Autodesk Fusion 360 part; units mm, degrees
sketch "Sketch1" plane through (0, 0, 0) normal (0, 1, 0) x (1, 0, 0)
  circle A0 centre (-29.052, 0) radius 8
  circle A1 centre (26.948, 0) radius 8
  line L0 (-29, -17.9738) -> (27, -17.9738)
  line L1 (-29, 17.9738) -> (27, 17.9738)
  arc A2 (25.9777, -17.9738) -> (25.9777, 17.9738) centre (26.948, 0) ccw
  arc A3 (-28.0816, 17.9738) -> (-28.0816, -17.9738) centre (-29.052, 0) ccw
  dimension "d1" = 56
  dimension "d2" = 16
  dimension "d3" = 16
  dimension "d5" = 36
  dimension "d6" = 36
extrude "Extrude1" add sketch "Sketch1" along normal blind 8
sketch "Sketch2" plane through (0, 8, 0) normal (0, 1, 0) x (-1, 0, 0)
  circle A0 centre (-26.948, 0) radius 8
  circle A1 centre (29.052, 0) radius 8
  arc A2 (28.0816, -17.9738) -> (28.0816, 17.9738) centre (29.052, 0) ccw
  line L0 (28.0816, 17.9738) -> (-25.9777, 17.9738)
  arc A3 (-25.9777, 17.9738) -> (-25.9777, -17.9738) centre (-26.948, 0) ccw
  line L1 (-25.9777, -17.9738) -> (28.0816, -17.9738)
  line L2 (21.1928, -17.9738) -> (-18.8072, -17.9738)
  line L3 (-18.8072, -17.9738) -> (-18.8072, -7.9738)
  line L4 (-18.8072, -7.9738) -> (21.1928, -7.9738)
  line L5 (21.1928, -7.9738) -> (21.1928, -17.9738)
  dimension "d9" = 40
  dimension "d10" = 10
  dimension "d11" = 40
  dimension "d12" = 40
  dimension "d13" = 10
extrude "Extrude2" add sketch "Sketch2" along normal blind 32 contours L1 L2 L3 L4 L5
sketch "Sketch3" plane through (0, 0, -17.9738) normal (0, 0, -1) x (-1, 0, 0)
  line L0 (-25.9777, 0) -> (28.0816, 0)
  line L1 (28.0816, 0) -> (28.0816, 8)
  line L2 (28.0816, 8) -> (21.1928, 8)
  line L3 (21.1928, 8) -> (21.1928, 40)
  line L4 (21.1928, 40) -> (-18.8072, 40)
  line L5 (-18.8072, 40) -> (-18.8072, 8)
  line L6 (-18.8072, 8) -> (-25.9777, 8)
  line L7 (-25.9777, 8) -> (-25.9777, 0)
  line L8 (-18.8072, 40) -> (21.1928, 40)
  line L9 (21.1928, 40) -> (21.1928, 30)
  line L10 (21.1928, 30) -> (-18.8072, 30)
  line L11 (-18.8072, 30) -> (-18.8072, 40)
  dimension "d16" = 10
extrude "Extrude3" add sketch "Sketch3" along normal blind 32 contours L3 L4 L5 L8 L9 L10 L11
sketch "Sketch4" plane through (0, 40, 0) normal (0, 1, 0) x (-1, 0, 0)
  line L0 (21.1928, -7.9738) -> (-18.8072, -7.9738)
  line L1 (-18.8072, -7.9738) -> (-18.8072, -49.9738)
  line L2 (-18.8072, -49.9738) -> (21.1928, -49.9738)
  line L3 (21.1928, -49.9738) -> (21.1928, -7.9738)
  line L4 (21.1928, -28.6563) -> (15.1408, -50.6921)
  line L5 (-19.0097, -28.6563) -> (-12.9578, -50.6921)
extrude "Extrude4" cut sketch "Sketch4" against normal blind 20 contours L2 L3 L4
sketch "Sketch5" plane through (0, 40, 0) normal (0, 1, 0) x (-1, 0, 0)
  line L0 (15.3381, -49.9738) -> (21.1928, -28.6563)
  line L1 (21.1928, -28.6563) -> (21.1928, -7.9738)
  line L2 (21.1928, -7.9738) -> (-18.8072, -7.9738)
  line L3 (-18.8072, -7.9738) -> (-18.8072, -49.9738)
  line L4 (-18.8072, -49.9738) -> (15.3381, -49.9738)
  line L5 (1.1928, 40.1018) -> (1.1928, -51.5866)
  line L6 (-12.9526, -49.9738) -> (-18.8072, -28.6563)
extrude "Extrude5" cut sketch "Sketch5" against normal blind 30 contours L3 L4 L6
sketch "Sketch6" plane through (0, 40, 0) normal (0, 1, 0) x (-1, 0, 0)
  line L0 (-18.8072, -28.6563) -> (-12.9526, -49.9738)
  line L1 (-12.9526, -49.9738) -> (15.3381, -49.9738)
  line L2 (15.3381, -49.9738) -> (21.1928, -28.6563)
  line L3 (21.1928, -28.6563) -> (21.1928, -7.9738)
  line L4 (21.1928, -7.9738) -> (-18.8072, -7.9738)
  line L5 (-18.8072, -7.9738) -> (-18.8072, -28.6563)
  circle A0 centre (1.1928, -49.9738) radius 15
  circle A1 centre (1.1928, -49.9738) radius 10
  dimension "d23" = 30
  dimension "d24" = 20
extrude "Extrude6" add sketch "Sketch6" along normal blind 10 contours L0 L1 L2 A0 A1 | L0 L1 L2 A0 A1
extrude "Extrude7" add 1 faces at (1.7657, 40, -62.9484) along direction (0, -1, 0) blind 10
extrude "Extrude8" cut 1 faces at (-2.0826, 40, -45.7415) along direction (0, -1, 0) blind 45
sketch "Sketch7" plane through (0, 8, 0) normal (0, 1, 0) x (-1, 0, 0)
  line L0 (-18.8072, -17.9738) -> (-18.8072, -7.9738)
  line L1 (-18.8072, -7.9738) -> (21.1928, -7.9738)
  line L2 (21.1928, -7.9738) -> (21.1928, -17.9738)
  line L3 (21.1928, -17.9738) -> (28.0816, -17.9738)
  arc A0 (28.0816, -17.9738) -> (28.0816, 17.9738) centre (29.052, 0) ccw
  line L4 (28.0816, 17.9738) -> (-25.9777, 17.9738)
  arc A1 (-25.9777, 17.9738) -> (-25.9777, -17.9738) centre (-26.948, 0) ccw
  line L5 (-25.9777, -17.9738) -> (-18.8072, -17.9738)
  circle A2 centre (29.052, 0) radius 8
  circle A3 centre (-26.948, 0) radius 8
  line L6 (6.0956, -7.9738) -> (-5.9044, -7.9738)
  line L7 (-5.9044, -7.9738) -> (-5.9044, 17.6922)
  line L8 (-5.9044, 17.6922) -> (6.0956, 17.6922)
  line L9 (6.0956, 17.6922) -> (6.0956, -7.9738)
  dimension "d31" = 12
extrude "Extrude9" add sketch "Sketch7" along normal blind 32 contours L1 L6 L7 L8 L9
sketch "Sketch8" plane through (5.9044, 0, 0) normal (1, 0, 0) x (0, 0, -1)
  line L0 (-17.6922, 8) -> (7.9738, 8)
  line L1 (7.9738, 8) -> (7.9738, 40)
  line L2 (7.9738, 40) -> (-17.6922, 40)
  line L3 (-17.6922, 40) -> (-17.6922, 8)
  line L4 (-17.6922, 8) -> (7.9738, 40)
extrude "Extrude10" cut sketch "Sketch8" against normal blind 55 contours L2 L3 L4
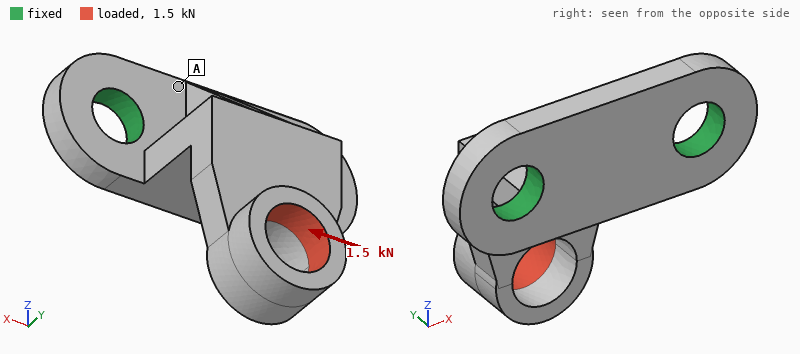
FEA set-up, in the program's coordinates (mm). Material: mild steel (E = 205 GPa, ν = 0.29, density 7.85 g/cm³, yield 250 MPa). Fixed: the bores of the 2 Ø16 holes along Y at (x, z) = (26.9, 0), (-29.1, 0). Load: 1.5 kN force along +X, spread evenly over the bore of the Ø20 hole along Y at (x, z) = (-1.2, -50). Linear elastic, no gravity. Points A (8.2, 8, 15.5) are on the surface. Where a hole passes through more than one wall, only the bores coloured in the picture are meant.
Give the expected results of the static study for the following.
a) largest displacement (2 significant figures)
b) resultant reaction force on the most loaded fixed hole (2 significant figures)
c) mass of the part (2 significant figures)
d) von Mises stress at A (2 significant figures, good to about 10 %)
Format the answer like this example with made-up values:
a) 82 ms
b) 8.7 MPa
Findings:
a) 55 µm
b) 2.1 kN
c) 430 g
d) 5.4 MPa
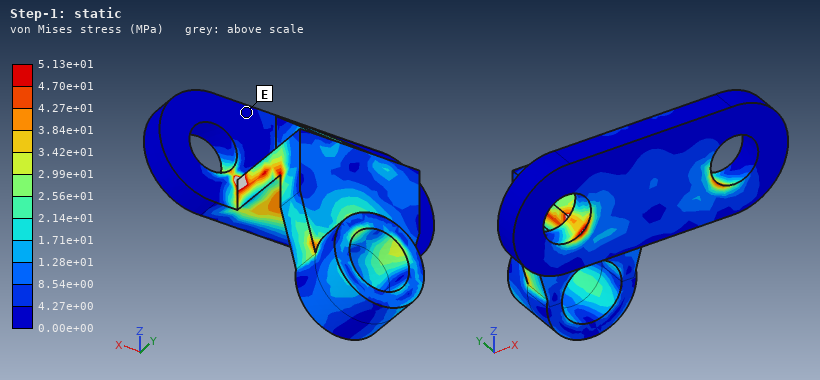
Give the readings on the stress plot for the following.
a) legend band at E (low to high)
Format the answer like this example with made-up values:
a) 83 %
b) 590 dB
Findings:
a) 0.00e+00 to 4.27e+00 MPa
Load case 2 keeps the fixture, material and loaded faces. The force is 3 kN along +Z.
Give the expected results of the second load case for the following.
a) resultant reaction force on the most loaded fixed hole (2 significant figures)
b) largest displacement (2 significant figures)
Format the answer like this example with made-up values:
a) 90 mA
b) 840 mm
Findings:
a) 1.6 kN
b) 0.18 mm
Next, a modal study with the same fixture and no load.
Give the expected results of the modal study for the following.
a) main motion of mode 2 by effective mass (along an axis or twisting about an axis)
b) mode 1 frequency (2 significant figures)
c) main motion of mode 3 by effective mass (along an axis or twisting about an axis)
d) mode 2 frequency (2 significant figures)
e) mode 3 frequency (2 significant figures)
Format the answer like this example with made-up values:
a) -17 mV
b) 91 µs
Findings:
a) along X
b) 2000 Hz
c) along Z
d) 3400 Hz
e) 5100 Hz
